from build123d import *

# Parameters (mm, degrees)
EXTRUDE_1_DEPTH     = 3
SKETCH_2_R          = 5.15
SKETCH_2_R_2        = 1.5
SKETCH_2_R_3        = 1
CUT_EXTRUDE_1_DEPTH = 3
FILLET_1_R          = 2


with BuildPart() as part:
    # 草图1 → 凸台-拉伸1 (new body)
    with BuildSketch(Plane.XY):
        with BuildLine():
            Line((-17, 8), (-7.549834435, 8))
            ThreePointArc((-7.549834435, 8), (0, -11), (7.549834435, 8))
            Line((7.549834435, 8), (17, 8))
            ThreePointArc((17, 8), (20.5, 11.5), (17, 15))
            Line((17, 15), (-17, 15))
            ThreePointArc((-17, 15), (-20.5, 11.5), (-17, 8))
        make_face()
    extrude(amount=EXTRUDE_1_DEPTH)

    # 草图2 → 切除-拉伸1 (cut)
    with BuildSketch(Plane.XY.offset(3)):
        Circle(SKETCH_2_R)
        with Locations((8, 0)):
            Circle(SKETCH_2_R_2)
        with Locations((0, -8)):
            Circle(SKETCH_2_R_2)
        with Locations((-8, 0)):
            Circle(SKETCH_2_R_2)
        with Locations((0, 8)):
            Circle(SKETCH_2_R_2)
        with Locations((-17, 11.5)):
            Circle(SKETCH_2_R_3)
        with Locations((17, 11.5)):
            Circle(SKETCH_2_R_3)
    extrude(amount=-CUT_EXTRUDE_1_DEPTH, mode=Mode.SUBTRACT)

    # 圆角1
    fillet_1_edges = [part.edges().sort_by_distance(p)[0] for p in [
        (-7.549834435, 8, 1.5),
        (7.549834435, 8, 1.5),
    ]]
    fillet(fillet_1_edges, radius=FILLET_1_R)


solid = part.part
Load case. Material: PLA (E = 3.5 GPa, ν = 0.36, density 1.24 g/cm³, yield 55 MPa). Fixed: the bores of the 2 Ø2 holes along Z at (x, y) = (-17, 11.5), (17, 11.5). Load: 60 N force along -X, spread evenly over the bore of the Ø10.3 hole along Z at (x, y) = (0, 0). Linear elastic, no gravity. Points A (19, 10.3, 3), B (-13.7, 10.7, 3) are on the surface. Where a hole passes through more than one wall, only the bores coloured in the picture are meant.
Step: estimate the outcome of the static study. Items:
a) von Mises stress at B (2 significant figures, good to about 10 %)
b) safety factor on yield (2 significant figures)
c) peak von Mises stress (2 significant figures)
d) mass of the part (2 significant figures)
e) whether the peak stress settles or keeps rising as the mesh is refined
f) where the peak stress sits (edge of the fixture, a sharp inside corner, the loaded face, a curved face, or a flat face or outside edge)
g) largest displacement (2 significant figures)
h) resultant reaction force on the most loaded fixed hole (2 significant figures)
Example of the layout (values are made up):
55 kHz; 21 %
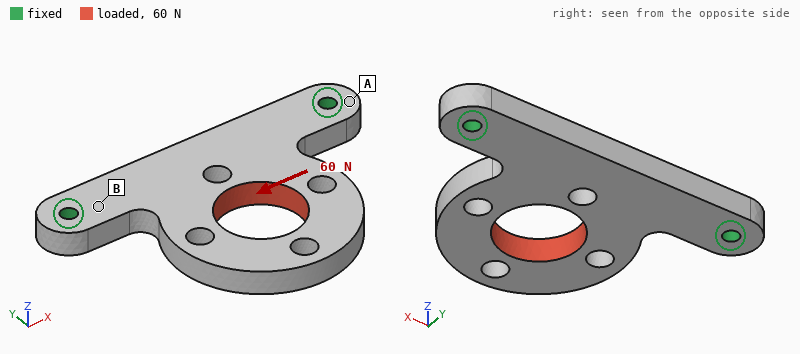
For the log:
3.7 MPa; 4.6; 12 MPa; 1.9 g; settles; a curved face; 71 µm; 38 N
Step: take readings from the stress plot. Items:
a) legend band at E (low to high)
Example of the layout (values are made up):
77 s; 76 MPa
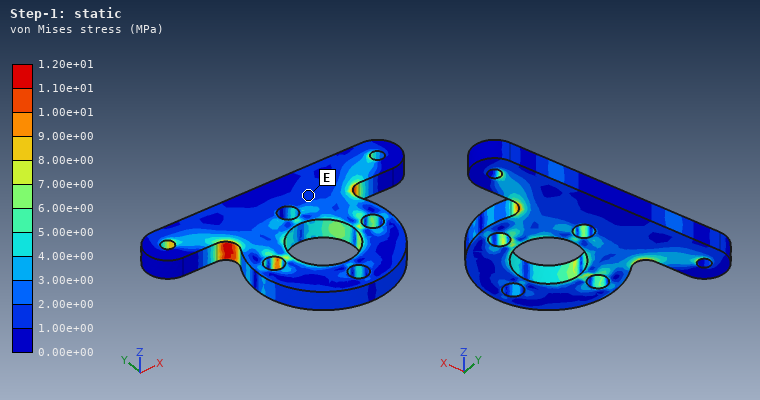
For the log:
1.00e+00 to 2.00e+00 MPa
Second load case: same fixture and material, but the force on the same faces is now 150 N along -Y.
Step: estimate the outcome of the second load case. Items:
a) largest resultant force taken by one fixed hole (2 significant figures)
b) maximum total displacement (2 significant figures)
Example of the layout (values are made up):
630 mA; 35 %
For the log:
82 N; 92 µm
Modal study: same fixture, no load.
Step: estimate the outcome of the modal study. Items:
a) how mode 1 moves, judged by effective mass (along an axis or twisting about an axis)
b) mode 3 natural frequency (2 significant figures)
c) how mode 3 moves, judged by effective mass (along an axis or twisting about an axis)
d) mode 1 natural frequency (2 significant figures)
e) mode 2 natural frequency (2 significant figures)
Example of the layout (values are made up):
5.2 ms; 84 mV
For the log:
along Z; 4100 Hz; along Z; 1100 Hz; 3600 Hz
